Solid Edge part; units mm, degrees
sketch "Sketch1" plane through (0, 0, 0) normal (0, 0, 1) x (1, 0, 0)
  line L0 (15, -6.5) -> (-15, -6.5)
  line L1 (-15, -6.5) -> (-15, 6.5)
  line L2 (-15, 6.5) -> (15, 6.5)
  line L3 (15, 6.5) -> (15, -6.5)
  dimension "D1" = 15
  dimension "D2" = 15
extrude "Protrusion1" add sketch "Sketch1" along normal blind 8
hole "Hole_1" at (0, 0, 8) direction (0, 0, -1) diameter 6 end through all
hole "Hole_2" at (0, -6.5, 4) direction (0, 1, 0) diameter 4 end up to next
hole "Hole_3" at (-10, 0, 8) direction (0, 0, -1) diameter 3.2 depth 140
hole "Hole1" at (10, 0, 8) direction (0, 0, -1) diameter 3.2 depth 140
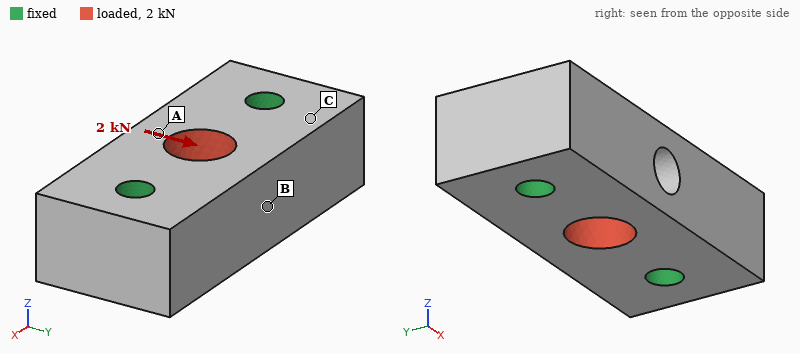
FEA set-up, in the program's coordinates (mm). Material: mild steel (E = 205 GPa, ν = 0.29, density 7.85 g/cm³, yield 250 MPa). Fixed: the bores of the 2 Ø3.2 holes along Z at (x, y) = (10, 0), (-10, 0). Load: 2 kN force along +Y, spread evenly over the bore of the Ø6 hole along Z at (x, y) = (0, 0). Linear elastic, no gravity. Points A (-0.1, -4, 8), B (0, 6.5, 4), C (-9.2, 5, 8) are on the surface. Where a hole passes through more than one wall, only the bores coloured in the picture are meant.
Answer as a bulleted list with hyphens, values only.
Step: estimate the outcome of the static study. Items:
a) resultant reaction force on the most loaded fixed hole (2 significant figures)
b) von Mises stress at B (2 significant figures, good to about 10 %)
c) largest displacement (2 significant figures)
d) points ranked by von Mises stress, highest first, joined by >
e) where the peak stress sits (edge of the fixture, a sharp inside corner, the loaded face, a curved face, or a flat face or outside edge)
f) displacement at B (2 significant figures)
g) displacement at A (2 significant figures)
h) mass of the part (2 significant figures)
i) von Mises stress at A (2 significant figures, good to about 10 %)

- 1.0 kN
- 40 MPa
- 2.0 µm
- B > A > C
- a curved face
- 1.8 µm
- 2.0 µm
- 21 g
- 18 MPa
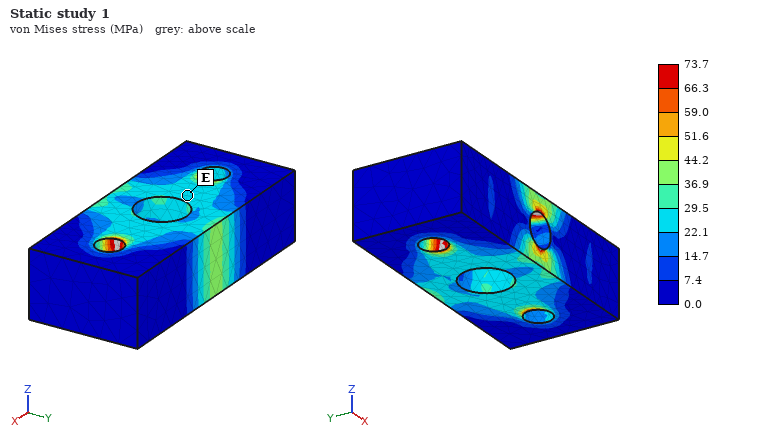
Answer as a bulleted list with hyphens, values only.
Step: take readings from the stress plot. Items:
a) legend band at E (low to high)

- 22.1 to 29.5 MPa
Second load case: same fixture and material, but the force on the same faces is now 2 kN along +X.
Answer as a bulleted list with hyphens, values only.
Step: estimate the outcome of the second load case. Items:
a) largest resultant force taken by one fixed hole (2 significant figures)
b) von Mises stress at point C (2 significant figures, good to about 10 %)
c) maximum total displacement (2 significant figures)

- 1.0 kN
- 4.2 MPa
- 0.72 µm
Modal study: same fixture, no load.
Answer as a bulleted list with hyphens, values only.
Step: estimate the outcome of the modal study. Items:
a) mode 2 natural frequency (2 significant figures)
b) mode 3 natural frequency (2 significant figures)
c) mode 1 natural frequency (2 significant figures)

- 62 kHz
- 64 kHz
- 60 kHz
